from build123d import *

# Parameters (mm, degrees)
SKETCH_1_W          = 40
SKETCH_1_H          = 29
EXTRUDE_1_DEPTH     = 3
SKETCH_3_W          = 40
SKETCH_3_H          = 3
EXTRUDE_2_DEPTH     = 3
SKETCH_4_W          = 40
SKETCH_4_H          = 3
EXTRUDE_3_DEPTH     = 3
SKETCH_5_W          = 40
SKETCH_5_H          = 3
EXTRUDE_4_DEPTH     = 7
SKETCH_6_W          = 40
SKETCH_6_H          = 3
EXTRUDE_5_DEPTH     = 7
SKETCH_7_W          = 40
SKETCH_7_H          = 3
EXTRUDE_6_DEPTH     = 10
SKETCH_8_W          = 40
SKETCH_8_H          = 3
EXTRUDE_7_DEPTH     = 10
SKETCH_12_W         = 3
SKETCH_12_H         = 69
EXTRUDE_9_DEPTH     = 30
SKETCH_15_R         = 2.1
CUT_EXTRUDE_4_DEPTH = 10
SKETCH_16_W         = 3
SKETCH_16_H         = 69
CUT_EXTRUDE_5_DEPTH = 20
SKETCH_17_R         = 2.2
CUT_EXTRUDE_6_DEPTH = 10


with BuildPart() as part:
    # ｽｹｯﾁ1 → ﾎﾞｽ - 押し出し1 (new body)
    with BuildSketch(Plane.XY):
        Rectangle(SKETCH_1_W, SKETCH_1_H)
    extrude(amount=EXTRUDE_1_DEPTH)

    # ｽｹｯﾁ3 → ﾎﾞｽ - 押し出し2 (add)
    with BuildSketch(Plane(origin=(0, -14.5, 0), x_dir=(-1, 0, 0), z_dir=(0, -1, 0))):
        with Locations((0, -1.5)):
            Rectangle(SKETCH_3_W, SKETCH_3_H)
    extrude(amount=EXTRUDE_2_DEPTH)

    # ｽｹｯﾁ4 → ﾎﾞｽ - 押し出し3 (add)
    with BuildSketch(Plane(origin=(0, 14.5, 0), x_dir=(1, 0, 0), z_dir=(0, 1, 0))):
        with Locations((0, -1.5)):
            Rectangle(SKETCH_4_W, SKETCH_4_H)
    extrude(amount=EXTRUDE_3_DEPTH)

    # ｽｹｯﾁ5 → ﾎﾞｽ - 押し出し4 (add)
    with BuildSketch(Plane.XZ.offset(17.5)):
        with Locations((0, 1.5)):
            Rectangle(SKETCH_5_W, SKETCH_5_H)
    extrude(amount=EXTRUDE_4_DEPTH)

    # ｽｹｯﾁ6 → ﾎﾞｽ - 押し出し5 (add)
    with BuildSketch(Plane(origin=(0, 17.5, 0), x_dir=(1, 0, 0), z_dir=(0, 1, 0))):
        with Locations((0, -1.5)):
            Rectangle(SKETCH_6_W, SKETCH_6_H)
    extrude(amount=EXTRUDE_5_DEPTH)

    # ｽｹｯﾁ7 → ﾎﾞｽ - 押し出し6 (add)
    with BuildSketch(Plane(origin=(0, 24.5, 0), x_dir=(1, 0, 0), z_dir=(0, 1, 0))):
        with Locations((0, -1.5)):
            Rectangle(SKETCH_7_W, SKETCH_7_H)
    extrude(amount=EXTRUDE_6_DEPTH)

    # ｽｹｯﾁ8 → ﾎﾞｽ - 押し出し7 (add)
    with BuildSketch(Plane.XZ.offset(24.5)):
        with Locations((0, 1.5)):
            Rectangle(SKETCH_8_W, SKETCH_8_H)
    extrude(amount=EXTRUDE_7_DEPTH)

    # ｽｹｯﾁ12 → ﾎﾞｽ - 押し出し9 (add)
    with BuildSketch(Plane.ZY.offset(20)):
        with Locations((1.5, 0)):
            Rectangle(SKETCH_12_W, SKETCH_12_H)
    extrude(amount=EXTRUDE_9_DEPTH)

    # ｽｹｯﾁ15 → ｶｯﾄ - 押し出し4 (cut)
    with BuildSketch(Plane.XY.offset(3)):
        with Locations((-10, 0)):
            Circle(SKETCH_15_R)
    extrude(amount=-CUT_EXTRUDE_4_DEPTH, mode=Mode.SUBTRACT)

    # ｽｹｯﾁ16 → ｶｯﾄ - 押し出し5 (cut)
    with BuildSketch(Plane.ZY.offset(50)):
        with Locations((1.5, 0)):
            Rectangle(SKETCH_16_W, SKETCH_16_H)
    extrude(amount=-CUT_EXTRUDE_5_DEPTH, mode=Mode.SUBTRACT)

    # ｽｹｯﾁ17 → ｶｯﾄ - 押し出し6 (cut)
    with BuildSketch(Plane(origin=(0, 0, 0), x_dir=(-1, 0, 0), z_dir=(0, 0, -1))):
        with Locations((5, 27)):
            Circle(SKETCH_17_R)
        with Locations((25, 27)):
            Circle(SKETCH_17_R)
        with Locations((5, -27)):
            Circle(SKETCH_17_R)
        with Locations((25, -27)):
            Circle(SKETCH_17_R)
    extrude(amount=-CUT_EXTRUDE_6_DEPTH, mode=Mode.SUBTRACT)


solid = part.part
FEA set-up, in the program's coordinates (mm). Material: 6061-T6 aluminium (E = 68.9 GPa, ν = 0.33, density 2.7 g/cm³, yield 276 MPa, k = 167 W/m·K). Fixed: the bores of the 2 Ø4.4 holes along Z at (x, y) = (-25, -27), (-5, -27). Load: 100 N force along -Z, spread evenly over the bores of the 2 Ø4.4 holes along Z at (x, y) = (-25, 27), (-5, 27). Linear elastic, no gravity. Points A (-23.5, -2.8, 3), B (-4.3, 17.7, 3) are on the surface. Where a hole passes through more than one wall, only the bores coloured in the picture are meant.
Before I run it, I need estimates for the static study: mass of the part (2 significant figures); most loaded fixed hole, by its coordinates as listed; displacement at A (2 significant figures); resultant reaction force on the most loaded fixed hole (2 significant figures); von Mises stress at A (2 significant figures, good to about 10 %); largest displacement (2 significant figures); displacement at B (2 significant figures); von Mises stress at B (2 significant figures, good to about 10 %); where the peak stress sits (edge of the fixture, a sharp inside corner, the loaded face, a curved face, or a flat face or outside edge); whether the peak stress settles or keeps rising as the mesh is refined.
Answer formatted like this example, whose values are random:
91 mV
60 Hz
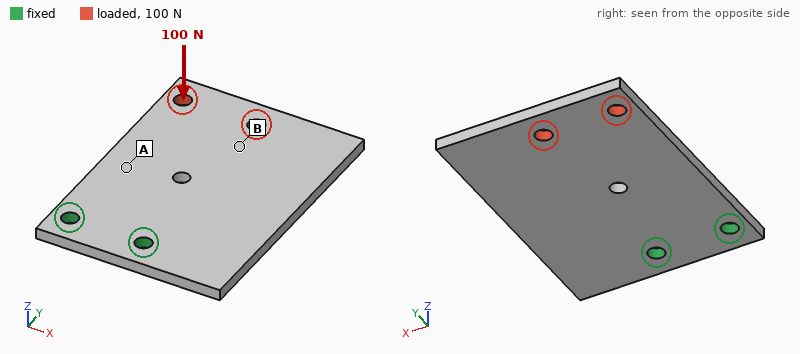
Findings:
27 g
(-5, -27)
0.19 mm
63 N
46 MPa
0.92 mm
0.53 mm
17 MPa
edge of the fixture
keeps rising
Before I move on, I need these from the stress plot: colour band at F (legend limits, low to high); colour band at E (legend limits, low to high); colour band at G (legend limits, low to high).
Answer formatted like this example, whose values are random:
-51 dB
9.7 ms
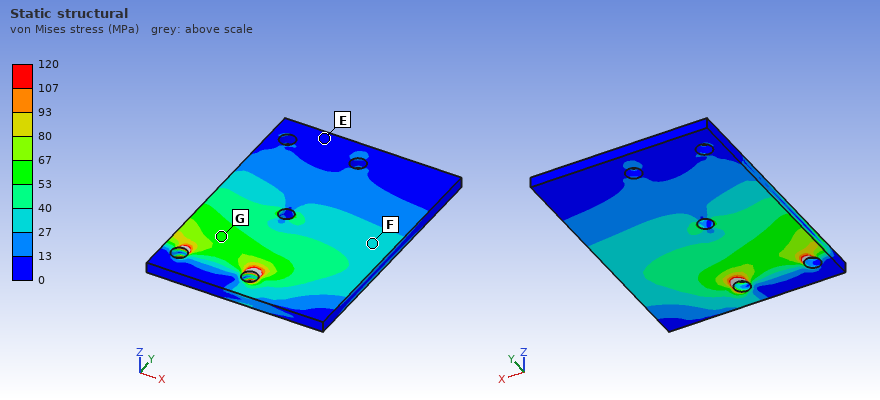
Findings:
27 to 40 MPa
0 to 13 MPa
53 to 67 MPa
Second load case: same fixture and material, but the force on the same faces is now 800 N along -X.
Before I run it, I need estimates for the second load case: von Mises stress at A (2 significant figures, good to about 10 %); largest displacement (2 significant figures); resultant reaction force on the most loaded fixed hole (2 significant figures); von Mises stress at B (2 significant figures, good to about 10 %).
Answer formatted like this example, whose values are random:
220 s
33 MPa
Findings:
23 MPa
93 µm
1.9 kN
14 MPa
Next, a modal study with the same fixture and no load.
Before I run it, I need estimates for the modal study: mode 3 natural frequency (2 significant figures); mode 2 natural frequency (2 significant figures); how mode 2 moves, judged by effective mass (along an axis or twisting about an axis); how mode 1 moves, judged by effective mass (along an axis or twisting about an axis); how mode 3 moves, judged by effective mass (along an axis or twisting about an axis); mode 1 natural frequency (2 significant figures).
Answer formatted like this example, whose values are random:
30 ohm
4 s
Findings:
3500 Hz
1600 Hz
twisting about Y
along Z
along Z
630 Hz
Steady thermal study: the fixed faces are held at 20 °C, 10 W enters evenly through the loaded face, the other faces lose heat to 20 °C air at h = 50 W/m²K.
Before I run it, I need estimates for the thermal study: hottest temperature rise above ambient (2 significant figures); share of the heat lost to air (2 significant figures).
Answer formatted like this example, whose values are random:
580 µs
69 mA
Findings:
23 K
34 %
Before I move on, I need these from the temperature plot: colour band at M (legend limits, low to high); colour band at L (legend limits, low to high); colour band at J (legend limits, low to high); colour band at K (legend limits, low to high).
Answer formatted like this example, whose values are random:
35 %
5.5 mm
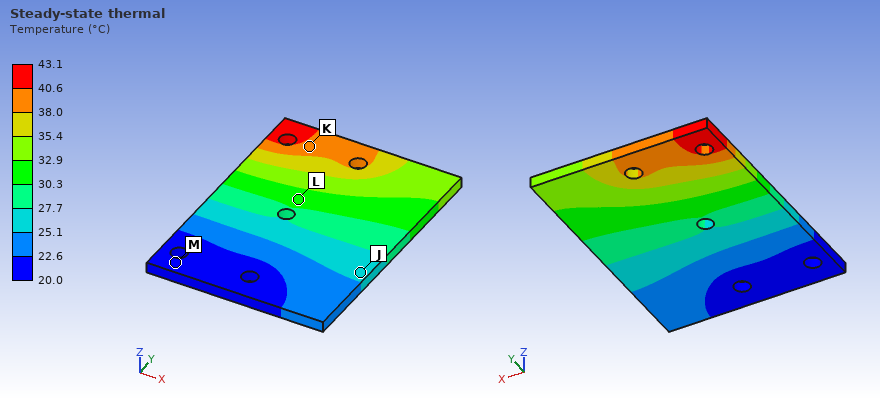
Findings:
20.0 to 22.6 °C
30.3 to 32.9 °C
25.1 to 27.7 °C
38.0 to 40.6 °C
